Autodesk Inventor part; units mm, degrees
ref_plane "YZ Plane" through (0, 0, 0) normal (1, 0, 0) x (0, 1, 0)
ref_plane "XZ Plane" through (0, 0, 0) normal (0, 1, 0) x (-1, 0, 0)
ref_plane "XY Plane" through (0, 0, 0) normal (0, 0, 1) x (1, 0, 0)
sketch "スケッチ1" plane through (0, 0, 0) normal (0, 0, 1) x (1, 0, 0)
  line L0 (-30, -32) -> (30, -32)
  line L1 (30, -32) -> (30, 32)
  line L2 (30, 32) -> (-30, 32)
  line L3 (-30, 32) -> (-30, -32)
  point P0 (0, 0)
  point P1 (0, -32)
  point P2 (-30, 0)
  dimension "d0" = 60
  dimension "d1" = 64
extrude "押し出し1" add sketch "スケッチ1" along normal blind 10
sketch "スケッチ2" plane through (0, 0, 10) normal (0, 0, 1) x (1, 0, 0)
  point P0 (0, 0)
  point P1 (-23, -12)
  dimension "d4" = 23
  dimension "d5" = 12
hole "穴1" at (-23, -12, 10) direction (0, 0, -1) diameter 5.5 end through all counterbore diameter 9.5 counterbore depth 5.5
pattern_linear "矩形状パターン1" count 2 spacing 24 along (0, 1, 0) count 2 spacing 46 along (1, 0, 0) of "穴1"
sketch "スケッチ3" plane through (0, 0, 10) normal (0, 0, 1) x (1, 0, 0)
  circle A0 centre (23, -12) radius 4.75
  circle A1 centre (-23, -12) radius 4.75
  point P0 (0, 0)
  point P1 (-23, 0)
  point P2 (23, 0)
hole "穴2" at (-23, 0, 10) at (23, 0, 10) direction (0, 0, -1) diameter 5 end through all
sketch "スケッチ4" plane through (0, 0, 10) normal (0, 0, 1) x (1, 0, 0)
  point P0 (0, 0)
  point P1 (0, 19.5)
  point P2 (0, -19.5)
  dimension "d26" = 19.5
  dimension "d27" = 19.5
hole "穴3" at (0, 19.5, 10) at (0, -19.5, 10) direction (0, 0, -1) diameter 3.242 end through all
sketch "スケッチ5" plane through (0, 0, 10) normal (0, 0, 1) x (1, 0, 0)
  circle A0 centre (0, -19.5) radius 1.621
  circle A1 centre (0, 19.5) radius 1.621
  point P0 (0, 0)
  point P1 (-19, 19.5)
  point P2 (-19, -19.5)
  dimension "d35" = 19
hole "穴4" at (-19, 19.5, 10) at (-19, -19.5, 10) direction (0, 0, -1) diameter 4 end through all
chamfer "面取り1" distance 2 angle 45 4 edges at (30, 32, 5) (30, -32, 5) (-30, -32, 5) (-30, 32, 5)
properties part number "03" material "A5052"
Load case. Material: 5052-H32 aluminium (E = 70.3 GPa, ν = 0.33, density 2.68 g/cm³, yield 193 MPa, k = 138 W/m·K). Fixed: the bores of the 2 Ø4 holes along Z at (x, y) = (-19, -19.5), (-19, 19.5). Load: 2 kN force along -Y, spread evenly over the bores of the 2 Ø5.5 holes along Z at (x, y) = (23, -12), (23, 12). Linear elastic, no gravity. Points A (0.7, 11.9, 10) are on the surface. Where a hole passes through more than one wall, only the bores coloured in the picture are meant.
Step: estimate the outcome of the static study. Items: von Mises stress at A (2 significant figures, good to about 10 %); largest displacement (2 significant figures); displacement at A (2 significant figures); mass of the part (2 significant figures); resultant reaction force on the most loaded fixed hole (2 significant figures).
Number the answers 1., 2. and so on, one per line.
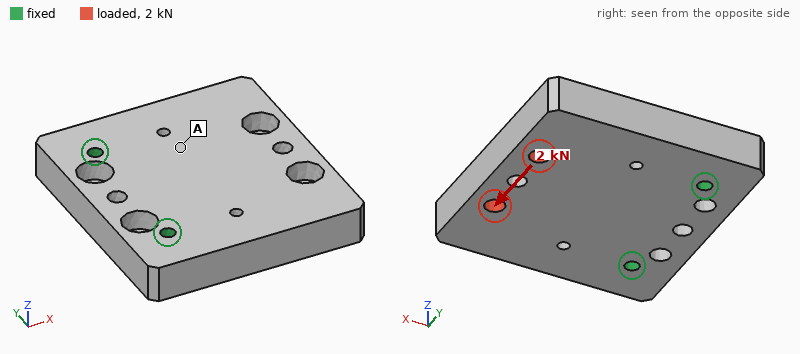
1. 6.2 MPa
2. 20 µm
3. 5.4 µm
4. 95 g
5. 2.3 kN
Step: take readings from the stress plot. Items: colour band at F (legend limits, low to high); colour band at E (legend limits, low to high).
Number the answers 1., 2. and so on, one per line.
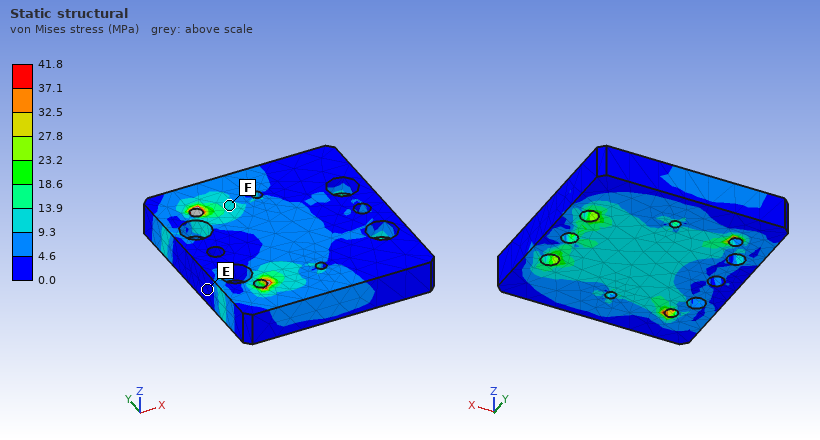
1. 9.3 to 13.9 MPa
2. 0.0 to 4.6 MPa
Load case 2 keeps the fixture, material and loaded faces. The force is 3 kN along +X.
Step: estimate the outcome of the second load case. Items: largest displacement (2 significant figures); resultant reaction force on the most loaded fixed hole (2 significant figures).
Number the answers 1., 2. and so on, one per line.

1. 35 µm
2. 1.5 kN
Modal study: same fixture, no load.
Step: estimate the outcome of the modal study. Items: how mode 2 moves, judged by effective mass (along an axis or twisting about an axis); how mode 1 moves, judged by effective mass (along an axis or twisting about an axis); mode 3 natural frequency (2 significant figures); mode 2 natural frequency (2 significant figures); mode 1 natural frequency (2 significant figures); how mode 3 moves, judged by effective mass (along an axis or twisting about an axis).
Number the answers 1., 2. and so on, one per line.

1. twisting about X
2. along Z
3. 10000 Hz
4. 5900 Hz
5. 2900 Hz
6. along Y
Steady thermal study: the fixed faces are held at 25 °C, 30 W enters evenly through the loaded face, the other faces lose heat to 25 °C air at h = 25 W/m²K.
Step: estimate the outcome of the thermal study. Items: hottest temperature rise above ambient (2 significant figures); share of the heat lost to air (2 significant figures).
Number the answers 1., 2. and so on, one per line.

1. 21 K
2. 7.8 %
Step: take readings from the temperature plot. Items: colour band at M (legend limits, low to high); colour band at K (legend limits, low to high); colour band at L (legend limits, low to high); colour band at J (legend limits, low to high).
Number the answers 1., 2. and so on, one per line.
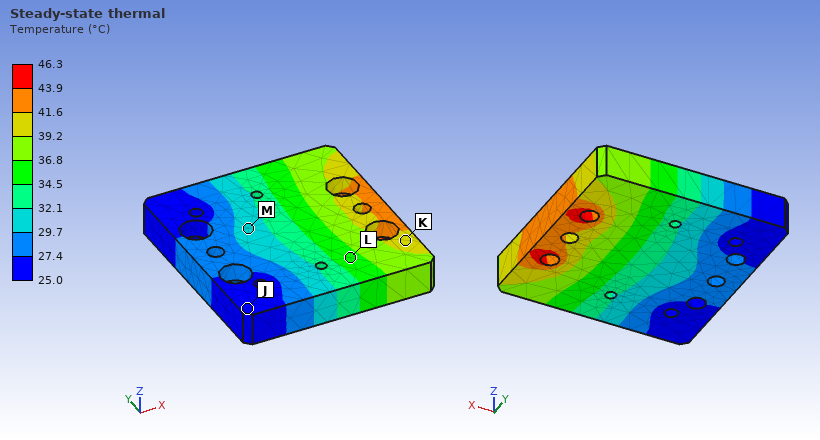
1. 29.7 to 32.1 °C
2. 39.2 to 41.6 °C
3. 34.5 to 36.8 °C
4. 25.0 to 27.4 °C
